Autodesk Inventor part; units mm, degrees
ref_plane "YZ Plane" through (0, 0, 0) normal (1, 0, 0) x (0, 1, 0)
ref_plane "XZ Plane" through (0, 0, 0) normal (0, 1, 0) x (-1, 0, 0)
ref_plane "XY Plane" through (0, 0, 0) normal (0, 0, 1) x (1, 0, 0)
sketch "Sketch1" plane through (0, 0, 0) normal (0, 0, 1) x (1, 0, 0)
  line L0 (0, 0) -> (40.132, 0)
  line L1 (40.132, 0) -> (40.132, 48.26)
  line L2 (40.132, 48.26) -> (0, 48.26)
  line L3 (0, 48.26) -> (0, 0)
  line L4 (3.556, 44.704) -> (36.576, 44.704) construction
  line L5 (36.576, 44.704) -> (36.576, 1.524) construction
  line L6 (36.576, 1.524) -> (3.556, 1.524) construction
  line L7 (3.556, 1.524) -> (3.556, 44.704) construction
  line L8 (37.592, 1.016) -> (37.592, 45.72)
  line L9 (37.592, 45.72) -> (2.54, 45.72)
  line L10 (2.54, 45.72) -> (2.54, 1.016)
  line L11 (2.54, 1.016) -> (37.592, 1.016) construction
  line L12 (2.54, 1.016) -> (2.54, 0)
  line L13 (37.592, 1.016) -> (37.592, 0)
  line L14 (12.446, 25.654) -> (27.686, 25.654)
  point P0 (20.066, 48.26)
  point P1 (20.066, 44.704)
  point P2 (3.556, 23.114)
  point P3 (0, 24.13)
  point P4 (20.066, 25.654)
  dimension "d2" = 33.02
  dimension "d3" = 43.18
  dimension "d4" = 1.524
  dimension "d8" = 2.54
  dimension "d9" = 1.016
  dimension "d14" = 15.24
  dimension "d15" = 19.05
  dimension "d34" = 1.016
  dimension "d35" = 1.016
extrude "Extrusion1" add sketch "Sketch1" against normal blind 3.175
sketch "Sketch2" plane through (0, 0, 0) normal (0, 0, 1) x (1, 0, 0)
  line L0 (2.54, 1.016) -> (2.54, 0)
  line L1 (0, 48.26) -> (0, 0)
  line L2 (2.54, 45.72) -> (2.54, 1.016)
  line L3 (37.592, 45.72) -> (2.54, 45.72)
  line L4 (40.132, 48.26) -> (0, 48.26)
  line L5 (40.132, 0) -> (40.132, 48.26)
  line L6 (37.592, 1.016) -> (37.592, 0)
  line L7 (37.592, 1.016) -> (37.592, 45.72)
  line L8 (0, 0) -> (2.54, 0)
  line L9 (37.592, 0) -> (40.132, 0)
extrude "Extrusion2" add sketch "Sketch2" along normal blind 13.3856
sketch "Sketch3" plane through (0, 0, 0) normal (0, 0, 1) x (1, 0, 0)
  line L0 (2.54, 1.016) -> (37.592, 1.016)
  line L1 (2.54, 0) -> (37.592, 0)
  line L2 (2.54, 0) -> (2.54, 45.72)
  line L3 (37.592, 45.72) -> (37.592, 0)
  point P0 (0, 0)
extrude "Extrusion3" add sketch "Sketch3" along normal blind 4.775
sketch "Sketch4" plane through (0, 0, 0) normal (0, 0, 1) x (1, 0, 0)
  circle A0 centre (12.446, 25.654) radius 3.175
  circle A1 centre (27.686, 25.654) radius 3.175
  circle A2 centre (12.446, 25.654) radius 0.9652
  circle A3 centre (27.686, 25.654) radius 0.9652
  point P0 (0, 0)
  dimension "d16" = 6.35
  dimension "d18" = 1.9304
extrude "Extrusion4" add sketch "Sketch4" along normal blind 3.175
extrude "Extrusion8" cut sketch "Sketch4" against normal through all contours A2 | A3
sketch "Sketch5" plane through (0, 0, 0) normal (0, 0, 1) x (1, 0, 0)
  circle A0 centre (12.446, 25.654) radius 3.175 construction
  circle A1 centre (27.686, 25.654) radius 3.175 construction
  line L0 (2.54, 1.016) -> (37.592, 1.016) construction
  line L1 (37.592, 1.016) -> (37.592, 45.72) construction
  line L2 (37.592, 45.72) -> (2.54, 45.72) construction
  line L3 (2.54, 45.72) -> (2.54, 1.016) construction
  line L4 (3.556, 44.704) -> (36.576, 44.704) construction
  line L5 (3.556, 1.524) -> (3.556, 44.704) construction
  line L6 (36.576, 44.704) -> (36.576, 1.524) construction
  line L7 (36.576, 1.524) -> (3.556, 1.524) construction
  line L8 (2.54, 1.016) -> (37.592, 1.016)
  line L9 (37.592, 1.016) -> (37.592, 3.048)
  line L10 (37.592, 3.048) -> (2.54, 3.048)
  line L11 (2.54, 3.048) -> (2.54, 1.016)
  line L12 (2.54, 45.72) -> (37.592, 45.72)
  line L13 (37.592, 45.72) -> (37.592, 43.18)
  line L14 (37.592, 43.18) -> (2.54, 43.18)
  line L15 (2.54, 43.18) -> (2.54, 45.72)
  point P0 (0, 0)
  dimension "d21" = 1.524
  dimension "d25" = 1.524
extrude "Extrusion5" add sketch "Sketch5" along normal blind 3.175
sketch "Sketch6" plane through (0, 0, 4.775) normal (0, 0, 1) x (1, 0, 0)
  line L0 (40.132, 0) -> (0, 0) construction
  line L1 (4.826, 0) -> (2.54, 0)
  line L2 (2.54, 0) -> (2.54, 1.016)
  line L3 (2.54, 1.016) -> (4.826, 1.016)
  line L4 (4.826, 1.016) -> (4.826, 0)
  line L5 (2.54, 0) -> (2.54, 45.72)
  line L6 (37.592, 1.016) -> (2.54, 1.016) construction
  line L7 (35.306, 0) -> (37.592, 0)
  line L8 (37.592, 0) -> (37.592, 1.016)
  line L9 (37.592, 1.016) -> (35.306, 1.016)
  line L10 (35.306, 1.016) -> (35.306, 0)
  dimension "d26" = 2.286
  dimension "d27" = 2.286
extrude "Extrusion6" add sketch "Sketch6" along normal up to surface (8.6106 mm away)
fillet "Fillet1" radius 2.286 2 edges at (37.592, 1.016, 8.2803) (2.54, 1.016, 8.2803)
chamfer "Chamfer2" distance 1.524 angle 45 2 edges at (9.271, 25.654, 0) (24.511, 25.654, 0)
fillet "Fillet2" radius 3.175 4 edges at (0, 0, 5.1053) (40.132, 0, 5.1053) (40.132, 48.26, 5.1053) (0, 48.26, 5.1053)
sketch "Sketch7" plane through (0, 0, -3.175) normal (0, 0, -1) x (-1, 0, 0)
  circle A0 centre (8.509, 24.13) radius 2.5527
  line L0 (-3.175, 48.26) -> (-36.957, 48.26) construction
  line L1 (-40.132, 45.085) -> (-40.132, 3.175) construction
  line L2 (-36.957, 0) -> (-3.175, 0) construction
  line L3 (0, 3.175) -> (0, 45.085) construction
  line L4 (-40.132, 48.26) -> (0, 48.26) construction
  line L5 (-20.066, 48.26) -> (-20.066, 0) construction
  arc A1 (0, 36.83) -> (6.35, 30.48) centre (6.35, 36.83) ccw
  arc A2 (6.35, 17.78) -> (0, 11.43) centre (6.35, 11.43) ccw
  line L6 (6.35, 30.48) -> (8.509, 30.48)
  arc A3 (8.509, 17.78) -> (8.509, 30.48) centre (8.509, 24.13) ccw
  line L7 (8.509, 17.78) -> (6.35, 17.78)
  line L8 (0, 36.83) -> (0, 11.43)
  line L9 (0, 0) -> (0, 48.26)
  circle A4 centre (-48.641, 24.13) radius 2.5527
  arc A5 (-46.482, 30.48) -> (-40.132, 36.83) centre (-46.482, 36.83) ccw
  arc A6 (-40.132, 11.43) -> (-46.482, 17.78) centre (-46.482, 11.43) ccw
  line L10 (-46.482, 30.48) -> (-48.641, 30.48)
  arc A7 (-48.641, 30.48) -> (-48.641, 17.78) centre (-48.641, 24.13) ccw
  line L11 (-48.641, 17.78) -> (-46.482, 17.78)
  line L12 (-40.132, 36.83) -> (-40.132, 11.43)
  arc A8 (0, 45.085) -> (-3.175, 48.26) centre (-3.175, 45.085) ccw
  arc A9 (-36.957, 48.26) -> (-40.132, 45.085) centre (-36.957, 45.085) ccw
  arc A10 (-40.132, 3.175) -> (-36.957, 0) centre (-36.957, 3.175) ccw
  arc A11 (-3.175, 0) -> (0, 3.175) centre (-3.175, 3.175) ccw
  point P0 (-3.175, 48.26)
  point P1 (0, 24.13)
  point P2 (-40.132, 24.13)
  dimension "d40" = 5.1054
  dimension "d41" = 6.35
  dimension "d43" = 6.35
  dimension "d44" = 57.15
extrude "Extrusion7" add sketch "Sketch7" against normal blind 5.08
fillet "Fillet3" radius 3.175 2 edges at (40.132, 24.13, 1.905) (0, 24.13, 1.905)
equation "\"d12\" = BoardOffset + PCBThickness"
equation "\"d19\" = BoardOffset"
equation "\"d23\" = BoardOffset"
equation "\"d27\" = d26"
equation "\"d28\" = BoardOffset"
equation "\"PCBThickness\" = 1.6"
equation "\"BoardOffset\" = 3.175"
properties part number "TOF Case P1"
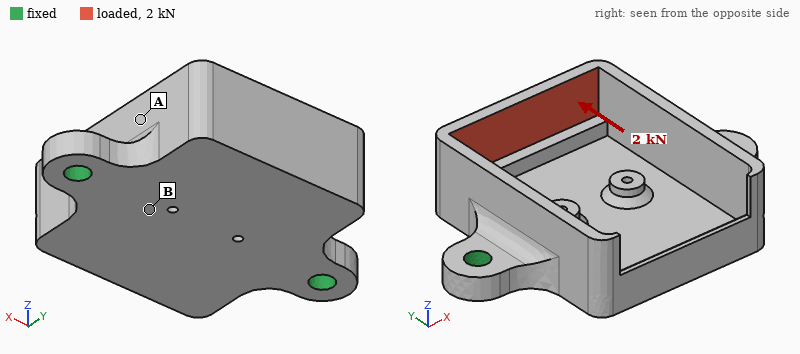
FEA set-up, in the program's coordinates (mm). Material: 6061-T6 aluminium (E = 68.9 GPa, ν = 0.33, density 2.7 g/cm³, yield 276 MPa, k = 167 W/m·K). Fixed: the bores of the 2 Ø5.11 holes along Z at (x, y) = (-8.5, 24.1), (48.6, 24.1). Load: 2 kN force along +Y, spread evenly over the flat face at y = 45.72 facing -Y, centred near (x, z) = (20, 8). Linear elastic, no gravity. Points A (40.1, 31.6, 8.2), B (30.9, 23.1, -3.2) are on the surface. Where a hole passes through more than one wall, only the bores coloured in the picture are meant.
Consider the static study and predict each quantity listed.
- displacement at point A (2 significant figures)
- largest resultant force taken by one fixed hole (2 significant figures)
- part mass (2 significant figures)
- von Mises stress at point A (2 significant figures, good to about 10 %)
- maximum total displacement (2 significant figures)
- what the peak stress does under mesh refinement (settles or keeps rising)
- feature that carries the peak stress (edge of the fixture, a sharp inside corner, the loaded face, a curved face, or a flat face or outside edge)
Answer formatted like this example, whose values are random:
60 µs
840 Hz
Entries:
0.060 mm
1.0 kN
36 g
41 MPa
0.29 mm
keeps rising
edge of the fixture
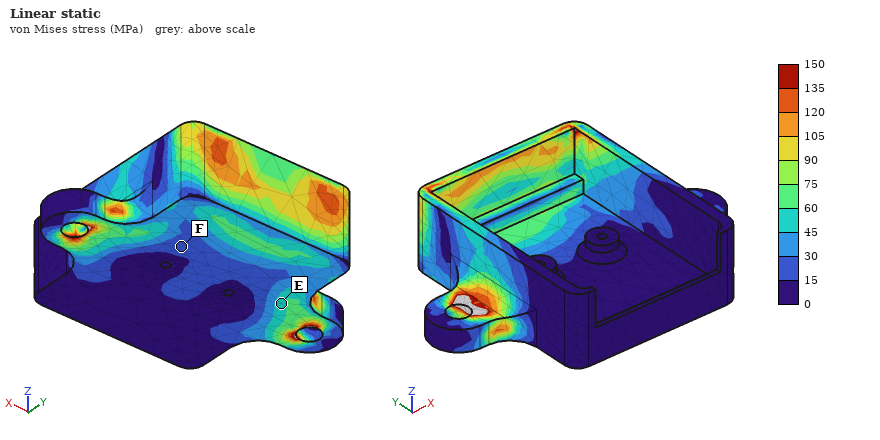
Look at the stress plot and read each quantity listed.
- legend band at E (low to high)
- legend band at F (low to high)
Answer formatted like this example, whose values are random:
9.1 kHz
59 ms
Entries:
45 to 60 MPa
15 to 30 MPa
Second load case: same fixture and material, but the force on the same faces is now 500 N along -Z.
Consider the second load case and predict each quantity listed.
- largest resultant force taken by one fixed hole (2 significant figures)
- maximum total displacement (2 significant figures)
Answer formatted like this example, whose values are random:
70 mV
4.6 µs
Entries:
260 N
96 µm
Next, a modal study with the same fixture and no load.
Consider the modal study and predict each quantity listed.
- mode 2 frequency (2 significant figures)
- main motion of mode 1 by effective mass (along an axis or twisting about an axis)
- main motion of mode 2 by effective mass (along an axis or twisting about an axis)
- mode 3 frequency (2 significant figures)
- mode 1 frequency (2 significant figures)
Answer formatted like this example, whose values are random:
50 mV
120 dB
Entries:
5800 Hz
twisting about X
along Z
6400 Hz
3300 Hz
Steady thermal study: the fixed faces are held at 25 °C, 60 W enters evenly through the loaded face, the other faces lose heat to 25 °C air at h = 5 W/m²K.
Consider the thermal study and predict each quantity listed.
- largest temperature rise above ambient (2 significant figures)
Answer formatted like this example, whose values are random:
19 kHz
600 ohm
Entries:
82 K
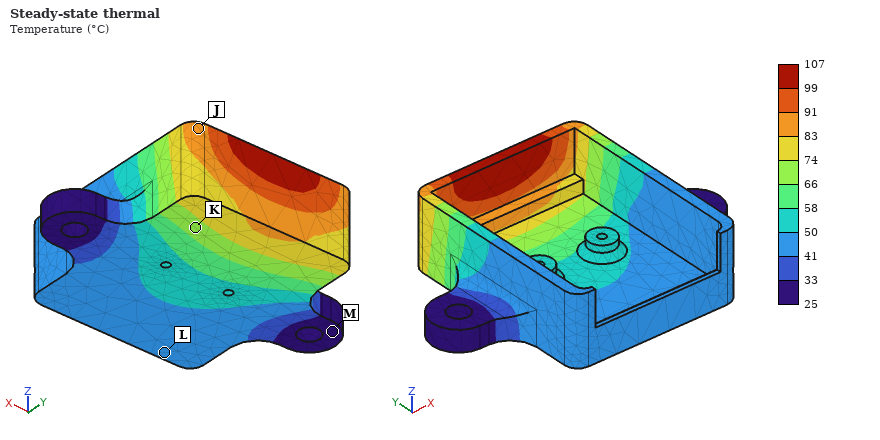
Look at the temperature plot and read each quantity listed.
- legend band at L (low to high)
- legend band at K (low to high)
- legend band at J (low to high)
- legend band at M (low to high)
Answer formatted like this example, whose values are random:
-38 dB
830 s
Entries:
41 to 50 °C
66 to 74 °C
83 to 91 °C
25 to 33 °C
